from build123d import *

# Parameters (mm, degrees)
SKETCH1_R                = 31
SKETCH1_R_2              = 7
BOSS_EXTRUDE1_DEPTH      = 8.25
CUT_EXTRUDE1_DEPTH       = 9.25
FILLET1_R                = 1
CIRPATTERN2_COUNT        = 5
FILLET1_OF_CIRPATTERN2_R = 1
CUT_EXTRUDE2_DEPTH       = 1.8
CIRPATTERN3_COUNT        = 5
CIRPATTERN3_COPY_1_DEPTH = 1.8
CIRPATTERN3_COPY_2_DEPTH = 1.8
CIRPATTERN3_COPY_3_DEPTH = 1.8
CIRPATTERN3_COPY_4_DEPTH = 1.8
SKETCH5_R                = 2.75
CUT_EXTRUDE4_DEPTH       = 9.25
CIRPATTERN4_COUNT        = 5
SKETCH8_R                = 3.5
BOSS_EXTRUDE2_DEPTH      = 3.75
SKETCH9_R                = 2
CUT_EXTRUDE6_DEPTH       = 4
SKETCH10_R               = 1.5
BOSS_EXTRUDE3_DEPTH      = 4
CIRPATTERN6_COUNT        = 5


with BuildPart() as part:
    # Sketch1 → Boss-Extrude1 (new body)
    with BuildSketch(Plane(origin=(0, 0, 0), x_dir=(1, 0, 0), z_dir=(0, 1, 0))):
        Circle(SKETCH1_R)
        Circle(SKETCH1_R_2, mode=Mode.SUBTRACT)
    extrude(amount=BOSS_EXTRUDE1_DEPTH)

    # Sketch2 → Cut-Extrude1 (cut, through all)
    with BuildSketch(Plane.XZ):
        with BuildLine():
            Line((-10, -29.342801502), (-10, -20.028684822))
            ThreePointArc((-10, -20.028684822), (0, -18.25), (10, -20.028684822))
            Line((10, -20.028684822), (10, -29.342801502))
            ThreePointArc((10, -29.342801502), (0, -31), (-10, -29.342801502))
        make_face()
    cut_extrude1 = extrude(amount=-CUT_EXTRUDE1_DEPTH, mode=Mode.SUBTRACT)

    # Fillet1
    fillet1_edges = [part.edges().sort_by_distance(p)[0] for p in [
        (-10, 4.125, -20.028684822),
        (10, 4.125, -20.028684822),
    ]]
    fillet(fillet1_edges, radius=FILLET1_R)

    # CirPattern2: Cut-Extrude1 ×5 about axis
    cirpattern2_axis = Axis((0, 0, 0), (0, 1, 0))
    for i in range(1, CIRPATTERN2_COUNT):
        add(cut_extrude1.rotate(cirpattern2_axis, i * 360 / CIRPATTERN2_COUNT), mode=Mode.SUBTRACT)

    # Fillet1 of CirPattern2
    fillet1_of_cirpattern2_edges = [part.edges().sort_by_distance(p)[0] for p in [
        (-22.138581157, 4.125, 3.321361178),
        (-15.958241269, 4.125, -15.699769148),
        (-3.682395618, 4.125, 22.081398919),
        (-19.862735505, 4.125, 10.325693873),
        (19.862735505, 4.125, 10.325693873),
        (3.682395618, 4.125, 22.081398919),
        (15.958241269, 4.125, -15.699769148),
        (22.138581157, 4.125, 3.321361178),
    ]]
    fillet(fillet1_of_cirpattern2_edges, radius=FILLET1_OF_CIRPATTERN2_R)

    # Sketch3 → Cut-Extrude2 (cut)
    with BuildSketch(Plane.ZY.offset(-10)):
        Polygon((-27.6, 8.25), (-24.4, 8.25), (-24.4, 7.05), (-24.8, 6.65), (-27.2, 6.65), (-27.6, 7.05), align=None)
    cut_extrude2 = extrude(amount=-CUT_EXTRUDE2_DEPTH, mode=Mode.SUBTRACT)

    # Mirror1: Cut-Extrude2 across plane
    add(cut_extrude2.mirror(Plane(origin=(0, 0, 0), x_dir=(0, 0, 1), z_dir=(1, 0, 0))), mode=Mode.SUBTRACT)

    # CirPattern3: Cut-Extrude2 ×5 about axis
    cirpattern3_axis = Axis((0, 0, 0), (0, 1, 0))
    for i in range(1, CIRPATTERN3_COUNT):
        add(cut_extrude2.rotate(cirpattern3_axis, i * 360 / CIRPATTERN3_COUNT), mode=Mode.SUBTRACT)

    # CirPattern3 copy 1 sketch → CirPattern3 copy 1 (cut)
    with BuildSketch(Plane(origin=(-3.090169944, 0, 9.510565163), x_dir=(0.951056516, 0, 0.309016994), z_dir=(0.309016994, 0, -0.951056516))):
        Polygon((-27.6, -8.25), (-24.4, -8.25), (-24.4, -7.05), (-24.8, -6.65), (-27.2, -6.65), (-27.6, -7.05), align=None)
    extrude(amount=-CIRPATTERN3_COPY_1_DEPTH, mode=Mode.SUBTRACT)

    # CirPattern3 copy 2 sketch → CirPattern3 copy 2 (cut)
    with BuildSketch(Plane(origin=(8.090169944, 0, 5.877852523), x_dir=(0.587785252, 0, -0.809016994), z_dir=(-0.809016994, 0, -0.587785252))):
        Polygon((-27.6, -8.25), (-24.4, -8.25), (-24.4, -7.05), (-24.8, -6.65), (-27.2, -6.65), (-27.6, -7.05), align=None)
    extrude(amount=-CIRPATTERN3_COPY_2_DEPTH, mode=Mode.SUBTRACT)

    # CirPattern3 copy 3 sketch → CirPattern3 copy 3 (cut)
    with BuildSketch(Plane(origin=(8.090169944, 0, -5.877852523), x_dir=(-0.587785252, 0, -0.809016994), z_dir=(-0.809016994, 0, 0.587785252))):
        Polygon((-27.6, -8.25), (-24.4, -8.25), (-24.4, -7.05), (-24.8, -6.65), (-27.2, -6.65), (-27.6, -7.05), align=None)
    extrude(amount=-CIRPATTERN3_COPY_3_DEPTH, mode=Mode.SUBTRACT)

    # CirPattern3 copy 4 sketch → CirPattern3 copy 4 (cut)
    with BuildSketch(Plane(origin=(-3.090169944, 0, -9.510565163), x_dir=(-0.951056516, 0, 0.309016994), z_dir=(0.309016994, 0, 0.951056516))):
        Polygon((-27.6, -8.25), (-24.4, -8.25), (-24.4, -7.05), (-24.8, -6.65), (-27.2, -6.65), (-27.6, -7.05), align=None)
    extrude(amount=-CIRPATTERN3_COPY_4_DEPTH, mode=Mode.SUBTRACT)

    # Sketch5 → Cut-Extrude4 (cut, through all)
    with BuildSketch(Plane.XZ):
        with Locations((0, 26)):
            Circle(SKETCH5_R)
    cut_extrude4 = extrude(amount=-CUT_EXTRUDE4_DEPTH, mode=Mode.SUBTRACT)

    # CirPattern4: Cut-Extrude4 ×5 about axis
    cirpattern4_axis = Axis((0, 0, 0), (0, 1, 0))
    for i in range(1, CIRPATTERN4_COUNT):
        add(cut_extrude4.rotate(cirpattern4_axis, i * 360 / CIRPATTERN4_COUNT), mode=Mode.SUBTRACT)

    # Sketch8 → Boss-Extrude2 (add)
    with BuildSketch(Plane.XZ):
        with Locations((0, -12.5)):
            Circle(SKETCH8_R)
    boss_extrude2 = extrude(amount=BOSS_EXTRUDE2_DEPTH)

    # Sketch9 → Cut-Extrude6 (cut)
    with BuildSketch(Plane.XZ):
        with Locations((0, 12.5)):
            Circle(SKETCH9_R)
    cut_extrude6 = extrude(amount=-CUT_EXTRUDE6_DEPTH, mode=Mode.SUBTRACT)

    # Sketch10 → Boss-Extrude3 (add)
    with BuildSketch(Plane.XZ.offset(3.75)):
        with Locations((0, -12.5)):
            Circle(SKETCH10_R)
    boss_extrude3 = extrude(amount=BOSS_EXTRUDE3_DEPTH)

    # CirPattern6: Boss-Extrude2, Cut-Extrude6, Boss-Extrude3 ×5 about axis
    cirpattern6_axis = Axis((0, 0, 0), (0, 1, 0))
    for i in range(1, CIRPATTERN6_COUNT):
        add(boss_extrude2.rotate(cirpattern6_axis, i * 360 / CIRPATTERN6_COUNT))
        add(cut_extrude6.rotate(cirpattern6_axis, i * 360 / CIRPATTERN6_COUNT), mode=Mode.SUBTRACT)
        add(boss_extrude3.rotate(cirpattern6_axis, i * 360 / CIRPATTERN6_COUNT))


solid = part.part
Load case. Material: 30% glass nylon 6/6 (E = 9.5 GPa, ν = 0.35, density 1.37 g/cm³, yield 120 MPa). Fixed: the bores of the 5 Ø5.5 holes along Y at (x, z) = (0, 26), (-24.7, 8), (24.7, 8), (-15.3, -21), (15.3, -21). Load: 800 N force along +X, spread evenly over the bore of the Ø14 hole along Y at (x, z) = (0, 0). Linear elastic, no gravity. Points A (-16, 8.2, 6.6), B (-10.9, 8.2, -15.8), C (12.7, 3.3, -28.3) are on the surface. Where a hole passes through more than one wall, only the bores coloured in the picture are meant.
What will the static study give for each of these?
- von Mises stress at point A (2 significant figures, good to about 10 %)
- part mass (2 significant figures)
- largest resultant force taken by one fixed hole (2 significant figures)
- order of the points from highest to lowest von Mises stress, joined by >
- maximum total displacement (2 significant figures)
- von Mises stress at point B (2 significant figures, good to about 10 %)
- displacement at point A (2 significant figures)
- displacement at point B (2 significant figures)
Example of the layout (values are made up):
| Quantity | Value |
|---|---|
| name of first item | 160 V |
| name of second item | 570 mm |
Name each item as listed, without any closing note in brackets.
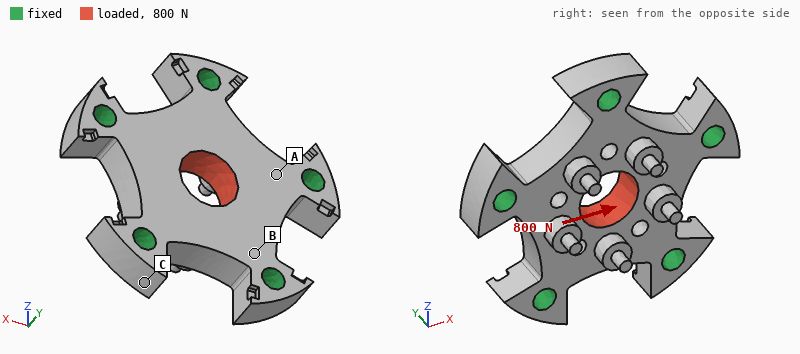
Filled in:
| Quantity | Value |
|---|---|
| von Mises stress at point A | 3.3 MPa |
| part mass | 19 g |
| largest resultant force taken by one fixed hole | 260 N |
| order of the points from highest to lowest von Mises stress, joined by > | A > B > C |
| maximum total displacement | 6.6 µm |
| von Mises stress at point B | 2.2 MPa |
| displacement at point A | 2.3 µm |
| displacement at point B | 1.6 µm |
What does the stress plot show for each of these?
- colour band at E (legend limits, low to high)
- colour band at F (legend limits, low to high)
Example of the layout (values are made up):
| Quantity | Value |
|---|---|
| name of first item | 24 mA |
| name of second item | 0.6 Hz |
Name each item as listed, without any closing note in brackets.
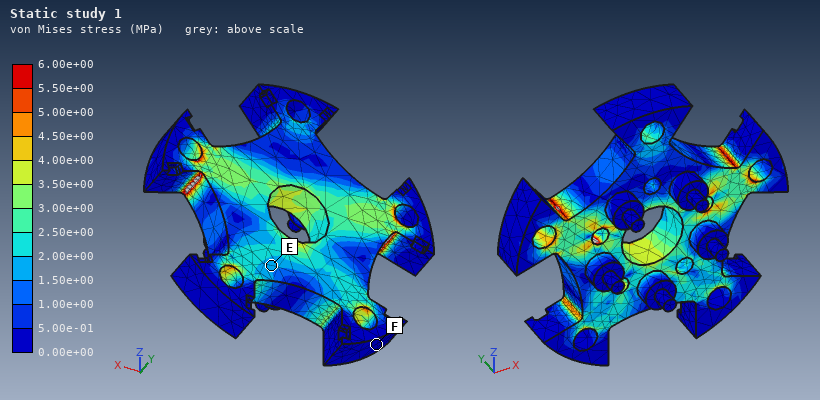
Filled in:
| Quantity | Value |
|---|---|
| colour band at E | 1.50e+00 to 2.00e+00 MPa |
| colour band at F | 0.00e+00 to 5.00e-01 MPa |
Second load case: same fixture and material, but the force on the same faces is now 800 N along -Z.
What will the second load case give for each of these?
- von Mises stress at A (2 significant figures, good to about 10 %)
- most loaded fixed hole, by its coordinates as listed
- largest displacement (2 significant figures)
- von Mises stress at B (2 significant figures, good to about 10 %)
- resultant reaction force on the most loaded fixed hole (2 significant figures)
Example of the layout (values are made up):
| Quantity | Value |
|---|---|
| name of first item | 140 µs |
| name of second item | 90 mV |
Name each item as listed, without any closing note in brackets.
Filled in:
| Quantity | Value |
|---|---|
| von Mises stress at A | 1.4 MPa |
| most loaded fixed hole, by its coordinates as listed | (0, 26) |
| largest displacement | 6.6 µm |
| von Mises stress at B | 2.8 MPa |
| resultant reaction force on the most loaded fixed hole | 270 N |
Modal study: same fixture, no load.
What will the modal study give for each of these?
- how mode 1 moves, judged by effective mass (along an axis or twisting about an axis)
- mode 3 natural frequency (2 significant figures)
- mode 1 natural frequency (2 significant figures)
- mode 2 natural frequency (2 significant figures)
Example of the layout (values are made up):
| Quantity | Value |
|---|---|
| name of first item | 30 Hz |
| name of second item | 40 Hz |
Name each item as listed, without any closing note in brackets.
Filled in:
| Quantity | Value |
|---|---|
| how mode 1 moves, judged by effective mass | along Y |
| mode 3 natural frequency | 16 kHz |
| mode 1 natural frequency | 10 kHz |
| mode 2 natural frequency | 16 kHz |
